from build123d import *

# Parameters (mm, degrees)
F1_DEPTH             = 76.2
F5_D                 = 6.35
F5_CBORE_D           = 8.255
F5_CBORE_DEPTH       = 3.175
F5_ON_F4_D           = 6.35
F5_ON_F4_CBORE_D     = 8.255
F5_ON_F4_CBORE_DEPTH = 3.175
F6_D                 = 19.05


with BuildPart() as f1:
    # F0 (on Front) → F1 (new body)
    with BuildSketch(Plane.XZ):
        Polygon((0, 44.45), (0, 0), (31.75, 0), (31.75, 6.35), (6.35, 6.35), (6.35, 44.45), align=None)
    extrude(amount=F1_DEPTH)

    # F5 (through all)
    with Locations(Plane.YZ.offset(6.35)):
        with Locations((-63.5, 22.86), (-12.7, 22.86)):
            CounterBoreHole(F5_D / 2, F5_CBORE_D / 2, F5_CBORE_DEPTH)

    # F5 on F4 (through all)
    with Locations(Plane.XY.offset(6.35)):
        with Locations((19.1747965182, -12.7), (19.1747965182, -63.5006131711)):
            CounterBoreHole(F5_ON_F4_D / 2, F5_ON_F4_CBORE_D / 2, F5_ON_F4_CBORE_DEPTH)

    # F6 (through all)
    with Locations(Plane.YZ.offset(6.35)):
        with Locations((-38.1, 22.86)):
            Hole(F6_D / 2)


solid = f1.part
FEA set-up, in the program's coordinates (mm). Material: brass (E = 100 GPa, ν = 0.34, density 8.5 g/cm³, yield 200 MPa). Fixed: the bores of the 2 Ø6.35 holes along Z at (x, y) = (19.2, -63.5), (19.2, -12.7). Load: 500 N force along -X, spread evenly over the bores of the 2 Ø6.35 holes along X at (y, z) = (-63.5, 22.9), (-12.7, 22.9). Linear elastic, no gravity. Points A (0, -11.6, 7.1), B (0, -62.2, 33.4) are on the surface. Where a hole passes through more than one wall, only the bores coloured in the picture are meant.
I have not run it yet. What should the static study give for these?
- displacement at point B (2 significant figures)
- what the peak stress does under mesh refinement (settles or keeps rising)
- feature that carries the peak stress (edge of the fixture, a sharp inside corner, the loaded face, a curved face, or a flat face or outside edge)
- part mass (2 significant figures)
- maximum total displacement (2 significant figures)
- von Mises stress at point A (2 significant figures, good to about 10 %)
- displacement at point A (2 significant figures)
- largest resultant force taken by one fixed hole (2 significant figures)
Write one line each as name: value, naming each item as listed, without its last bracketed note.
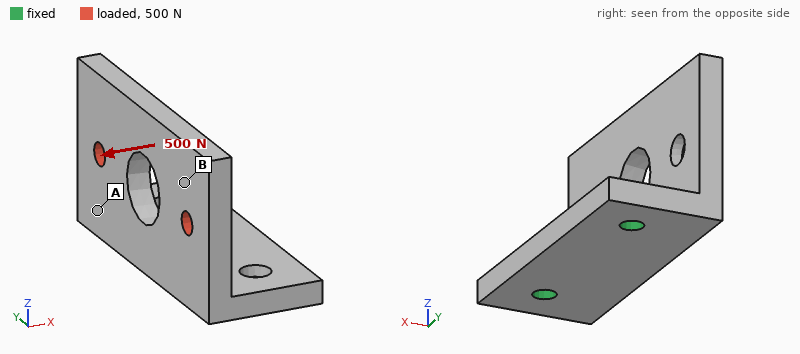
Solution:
displacement at point B: 67 µm
what the peak stress does under mesh refinement: keeps rising
feature that carries the peak stress: edge of the fixture
part mass: 260 g
maximum total displacement: 91 µm
von Mises stress at point A: 14 MPa
displacement at point A: 25 µm
largest resultant force taken by one fixed hole: 250 N
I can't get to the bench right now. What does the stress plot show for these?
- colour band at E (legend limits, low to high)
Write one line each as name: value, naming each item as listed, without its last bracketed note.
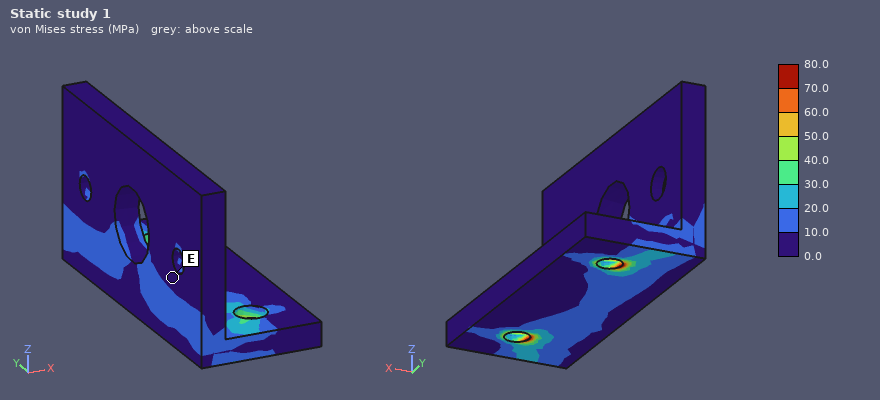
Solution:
colour band at E: 0.0 to 10.0 MPa
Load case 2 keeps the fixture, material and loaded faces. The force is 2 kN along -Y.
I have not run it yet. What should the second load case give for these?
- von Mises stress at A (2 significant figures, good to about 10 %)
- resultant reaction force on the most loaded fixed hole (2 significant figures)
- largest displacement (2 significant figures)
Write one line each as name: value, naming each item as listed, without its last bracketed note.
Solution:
von Mises stress at A: 10 MPa
resultant reaction force on the most loaded fixed hole: 1.4 kN
largest displacement: 45 µm
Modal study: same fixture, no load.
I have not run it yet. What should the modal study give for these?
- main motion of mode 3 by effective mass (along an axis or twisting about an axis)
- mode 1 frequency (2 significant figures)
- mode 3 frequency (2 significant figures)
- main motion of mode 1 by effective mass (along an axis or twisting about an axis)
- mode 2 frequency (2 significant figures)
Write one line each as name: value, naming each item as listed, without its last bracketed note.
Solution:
main motion of mode 3 by effective mass: along Y
mode 1 frequency: 1100 Hz
mode 3 frequency: 3600 Hz
main motion of mode 1 by effective mass: along X
mode 2 frequency: 2100 Hz
